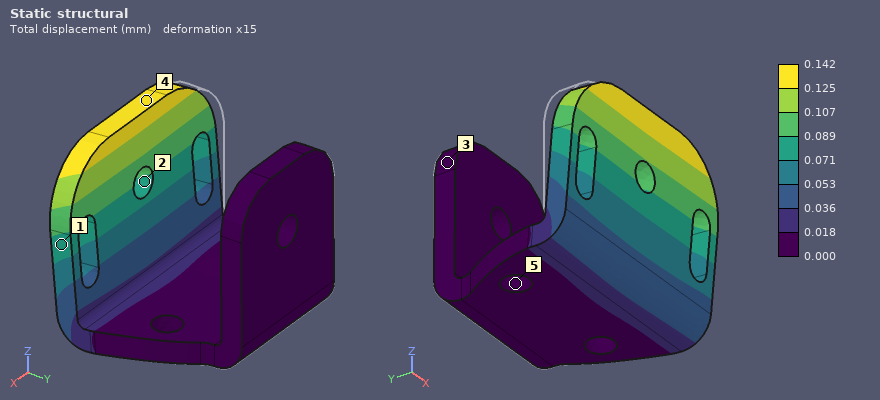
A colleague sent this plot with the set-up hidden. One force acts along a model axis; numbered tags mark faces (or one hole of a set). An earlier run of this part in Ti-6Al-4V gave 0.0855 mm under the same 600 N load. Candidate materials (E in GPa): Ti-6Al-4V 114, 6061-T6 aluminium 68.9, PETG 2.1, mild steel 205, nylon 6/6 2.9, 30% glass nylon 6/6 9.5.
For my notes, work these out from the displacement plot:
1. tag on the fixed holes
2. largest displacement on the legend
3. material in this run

5
0.142 mm
6061-T6 aluminium
